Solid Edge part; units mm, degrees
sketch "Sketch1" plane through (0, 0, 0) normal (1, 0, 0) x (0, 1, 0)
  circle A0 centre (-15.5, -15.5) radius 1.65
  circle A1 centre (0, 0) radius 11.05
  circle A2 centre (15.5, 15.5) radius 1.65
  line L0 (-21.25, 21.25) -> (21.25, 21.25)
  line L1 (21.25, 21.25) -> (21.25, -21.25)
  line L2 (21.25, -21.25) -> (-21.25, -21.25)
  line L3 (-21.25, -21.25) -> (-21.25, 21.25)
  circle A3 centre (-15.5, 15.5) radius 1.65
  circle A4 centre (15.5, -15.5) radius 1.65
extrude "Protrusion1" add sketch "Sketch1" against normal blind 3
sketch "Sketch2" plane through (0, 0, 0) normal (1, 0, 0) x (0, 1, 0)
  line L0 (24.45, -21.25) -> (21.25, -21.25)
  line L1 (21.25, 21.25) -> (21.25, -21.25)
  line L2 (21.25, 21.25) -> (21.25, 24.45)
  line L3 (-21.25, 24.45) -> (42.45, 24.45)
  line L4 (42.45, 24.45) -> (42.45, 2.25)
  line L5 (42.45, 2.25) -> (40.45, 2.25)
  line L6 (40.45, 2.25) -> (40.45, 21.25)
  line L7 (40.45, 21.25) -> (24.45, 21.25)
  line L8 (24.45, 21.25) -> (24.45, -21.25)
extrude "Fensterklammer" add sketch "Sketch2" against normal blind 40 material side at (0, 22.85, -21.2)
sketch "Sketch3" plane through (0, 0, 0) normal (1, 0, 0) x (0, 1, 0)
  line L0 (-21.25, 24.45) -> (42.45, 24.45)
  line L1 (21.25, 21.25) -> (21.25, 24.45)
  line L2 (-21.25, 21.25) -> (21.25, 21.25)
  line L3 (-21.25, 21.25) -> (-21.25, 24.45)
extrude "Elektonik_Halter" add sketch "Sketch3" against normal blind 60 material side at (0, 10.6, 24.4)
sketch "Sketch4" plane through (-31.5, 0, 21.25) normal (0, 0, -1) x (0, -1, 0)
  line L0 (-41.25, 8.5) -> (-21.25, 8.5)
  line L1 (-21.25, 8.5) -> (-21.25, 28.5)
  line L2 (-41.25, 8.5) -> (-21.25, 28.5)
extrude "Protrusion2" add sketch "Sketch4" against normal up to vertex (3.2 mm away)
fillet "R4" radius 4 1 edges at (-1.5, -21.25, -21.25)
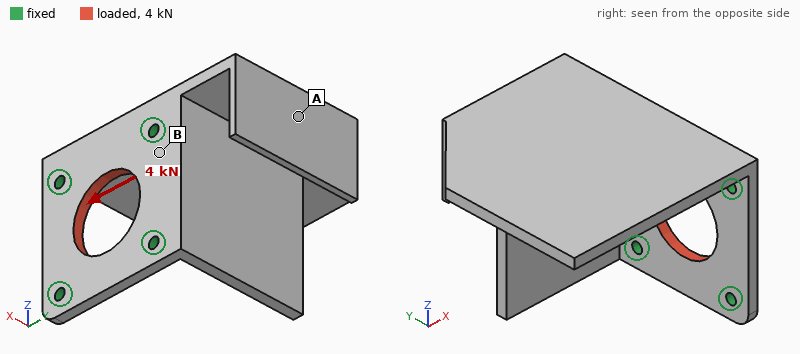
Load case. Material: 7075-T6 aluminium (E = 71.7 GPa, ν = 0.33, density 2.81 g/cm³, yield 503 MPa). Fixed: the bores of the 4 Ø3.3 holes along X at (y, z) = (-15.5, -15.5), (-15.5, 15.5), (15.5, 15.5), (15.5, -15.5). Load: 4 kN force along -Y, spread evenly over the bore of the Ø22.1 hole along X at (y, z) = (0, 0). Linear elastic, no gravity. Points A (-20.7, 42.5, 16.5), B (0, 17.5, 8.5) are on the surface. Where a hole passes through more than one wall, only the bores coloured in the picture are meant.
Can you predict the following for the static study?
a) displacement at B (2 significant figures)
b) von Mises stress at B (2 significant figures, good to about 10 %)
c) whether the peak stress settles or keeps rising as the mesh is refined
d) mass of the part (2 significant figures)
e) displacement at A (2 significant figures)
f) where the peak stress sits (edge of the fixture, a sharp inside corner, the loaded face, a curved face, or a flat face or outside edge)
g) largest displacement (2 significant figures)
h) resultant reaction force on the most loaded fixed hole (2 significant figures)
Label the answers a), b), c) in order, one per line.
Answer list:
a) 4.3 µm
b) 20 MPa
c) keeps rising
d) 64 g
e) 2.0 µm
f) edge of the fixture
g) 12 µm
h) 1.0 kN
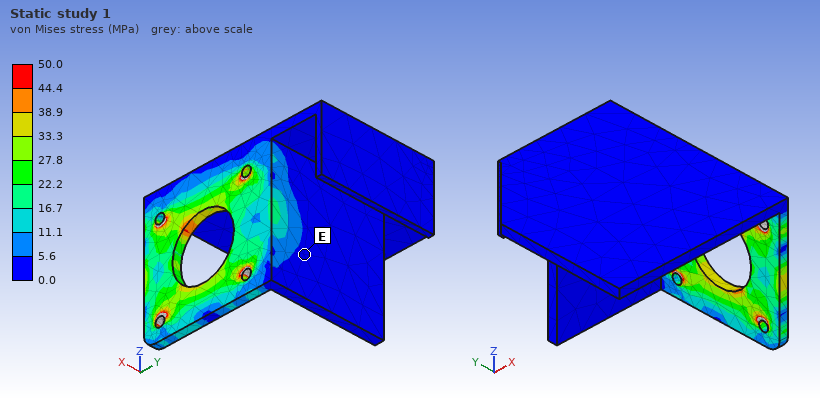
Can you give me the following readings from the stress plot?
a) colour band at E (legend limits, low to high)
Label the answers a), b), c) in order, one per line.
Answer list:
a) 0.0 to 5.6 MPa
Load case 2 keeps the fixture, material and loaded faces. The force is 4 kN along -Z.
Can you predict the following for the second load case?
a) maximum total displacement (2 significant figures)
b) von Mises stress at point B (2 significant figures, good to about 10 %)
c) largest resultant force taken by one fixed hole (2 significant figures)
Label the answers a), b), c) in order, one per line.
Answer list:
a) 12 µm
b) 16 MPa
c) 1.0 kN
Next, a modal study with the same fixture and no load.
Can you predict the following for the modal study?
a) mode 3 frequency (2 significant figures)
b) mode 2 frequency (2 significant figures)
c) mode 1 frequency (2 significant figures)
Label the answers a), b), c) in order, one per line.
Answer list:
a) 2700 Hz
b) 2200 Hz
c) 1300 Hz
